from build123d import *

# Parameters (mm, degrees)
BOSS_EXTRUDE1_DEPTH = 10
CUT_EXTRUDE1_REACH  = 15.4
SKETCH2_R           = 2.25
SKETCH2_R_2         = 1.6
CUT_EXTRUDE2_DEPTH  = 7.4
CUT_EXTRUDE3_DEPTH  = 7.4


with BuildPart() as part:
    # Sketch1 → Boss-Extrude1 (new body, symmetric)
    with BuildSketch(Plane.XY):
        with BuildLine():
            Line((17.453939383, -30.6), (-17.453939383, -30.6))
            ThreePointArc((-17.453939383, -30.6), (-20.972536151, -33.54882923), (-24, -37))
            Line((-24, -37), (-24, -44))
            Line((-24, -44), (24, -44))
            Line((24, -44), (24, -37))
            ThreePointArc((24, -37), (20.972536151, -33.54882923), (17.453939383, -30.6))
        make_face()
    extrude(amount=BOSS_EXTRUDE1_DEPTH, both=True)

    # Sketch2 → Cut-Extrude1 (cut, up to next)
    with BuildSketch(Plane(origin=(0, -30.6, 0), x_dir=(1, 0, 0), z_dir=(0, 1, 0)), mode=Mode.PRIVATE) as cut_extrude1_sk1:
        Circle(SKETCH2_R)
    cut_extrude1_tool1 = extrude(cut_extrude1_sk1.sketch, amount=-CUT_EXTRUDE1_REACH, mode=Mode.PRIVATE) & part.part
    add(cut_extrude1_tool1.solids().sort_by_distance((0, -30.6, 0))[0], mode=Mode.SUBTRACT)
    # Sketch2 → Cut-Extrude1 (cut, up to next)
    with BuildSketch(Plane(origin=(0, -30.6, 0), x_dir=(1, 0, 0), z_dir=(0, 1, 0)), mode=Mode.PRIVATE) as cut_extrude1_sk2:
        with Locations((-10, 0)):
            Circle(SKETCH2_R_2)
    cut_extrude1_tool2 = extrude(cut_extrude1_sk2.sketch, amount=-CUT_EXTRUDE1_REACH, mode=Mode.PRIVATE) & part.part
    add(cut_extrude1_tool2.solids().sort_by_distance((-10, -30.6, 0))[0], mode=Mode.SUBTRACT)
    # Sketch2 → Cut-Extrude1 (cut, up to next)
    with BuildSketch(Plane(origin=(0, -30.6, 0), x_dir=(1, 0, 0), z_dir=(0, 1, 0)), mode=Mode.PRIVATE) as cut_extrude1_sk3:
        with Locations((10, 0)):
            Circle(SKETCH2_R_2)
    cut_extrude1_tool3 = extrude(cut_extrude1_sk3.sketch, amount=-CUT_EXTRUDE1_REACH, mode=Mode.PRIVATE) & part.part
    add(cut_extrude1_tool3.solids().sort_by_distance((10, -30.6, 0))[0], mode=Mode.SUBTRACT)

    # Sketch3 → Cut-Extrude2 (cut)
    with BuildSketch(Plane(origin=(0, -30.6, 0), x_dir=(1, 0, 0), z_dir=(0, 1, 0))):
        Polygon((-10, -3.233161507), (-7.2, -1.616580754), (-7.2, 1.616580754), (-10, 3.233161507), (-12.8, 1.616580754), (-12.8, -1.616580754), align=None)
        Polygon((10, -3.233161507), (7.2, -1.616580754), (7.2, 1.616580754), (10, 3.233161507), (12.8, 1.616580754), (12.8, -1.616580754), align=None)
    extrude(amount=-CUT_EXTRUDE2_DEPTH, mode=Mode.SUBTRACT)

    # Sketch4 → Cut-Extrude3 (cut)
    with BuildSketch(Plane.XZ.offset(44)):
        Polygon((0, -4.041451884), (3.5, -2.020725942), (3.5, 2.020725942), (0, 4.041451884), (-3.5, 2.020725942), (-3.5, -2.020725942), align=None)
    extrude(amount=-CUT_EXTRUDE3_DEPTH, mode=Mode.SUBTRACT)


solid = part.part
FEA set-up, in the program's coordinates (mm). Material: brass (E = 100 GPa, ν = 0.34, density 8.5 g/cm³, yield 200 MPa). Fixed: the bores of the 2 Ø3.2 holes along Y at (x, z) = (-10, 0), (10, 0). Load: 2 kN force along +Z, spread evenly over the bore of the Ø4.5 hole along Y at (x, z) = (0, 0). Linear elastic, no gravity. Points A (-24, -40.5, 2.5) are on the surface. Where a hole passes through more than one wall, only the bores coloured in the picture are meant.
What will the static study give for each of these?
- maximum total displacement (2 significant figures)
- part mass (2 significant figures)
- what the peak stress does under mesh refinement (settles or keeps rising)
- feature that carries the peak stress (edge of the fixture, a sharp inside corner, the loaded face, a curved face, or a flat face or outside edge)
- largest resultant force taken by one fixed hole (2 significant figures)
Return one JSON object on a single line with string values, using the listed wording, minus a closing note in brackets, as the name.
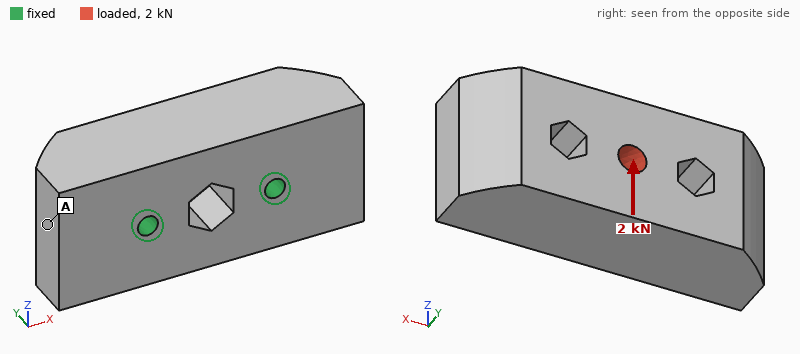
{"maximum total displacement": "12 µm", "part mass": "95 g", "what the peak stress does under mesh refinement": "keeps rising", "feature that carries the peak stress": "edge of the fixture", "largest resultant force taken by one fixed hole": "1.0 kN"}
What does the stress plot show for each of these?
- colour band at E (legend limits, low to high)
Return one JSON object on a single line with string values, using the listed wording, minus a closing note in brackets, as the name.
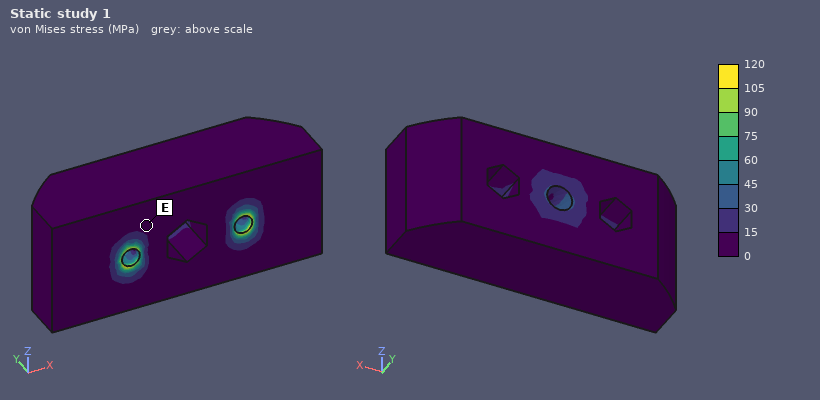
{"colour band at E": "0 to 15 MPa"}
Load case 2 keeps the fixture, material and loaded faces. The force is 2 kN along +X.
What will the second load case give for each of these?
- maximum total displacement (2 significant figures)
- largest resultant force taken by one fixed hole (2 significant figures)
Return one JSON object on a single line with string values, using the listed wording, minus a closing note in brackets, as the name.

{"maximum total displacement": "3.6 µm", "largest resultant force taken by one fixed hole": "1.2 kN"}
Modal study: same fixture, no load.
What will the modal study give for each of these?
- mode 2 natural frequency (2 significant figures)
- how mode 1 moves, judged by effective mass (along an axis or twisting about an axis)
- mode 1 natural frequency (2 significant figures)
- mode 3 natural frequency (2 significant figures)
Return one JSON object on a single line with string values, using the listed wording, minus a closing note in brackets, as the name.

{"mode 2 natural frequency": "14 kHz", "how mode 1 moves, judged by effective mass": "along Z", "mode 1 natural frequency": "9500 Hz", "mode 3 natural frequency": "14 kHz"}
